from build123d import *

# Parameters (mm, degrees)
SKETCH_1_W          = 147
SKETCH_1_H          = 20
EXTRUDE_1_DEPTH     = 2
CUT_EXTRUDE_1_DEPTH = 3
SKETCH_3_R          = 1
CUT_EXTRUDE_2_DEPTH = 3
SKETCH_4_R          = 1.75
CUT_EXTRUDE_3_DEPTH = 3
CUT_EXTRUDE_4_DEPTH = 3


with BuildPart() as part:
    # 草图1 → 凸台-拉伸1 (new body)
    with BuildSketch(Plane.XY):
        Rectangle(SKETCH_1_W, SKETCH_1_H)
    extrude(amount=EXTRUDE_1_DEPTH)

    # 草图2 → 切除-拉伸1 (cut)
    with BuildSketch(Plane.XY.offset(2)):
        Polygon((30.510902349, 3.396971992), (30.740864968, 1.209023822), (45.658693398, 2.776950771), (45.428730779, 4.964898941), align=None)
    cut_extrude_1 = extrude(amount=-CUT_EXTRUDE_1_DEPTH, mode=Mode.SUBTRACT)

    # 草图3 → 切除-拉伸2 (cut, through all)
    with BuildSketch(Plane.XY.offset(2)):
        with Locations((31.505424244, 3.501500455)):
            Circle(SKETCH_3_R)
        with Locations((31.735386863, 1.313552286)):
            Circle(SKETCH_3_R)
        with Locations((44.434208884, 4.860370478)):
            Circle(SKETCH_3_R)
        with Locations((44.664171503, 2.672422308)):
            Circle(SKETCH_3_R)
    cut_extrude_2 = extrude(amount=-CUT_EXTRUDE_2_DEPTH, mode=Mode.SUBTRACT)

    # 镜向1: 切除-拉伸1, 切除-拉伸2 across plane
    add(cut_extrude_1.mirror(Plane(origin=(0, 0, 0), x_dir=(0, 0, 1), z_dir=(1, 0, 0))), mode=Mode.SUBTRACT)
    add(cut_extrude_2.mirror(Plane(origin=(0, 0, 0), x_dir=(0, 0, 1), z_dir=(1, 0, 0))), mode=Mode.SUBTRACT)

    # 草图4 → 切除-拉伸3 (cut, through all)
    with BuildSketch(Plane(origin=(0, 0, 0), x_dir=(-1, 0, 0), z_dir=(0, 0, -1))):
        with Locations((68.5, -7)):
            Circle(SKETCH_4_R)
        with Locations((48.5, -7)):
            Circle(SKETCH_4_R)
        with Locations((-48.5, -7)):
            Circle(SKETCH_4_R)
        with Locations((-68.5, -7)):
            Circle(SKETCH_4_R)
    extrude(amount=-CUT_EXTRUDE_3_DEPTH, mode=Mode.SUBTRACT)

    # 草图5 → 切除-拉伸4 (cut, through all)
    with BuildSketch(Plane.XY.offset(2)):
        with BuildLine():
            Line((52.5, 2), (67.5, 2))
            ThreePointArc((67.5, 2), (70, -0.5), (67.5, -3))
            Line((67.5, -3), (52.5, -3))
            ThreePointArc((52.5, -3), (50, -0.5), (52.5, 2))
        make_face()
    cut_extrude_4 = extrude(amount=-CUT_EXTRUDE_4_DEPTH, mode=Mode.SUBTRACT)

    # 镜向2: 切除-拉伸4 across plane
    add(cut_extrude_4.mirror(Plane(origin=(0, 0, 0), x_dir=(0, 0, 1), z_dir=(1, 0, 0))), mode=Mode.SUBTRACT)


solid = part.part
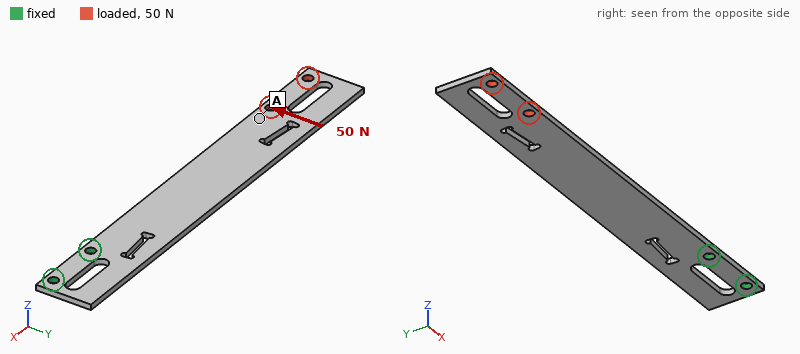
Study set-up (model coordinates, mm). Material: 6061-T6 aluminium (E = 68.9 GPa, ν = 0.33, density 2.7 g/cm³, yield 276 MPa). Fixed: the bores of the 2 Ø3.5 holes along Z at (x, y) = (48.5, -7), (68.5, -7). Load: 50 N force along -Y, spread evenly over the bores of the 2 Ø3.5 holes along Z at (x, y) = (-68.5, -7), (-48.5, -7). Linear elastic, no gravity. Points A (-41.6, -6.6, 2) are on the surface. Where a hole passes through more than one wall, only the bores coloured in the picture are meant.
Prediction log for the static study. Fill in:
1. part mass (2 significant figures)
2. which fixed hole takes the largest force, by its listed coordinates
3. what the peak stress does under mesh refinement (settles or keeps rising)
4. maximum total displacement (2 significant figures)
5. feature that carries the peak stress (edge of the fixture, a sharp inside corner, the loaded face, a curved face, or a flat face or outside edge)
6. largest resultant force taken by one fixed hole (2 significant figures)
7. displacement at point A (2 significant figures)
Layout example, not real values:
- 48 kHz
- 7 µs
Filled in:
- 14 g
- (48.5, -7)
- keeps rising
- 0.47 mm
- edge of the fixture
- 250 N
- 0.31 mm
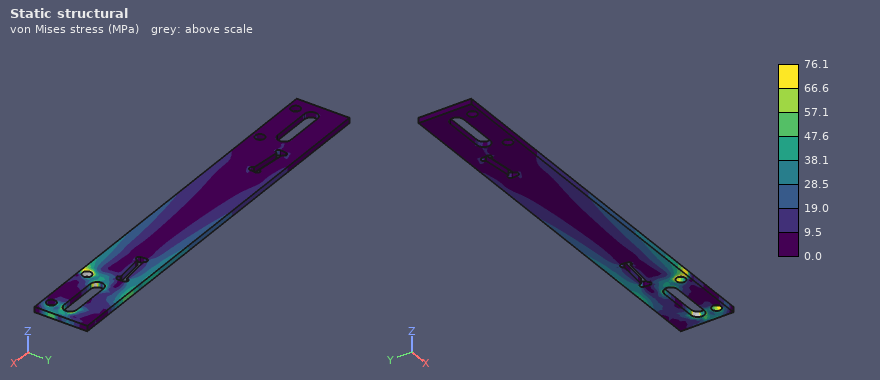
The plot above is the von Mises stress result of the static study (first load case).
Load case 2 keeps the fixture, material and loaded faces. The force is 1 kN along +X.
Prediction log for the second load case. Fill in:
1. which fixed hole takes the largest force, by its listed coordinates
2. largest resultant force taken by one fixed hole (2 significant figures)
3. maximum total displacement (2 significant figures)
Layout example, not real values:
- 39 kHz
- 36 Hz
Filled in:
- (48.5, -7)
- 980 N
- 0.56 mm
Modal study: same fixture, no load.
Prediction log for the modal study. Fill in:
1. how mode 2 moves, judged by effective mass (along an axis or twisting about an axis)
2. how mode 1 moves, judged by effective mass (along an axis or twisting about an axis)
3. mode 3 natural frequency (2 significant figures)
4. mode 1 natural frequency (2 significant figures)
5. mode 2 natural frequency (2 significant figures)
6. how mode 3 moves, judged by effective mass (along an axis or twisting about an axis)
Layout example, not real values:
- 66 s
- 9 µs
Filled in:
- along Z
- along Z
- 860 Hz
- 110 Hz
- 670 Hz
- along Y
